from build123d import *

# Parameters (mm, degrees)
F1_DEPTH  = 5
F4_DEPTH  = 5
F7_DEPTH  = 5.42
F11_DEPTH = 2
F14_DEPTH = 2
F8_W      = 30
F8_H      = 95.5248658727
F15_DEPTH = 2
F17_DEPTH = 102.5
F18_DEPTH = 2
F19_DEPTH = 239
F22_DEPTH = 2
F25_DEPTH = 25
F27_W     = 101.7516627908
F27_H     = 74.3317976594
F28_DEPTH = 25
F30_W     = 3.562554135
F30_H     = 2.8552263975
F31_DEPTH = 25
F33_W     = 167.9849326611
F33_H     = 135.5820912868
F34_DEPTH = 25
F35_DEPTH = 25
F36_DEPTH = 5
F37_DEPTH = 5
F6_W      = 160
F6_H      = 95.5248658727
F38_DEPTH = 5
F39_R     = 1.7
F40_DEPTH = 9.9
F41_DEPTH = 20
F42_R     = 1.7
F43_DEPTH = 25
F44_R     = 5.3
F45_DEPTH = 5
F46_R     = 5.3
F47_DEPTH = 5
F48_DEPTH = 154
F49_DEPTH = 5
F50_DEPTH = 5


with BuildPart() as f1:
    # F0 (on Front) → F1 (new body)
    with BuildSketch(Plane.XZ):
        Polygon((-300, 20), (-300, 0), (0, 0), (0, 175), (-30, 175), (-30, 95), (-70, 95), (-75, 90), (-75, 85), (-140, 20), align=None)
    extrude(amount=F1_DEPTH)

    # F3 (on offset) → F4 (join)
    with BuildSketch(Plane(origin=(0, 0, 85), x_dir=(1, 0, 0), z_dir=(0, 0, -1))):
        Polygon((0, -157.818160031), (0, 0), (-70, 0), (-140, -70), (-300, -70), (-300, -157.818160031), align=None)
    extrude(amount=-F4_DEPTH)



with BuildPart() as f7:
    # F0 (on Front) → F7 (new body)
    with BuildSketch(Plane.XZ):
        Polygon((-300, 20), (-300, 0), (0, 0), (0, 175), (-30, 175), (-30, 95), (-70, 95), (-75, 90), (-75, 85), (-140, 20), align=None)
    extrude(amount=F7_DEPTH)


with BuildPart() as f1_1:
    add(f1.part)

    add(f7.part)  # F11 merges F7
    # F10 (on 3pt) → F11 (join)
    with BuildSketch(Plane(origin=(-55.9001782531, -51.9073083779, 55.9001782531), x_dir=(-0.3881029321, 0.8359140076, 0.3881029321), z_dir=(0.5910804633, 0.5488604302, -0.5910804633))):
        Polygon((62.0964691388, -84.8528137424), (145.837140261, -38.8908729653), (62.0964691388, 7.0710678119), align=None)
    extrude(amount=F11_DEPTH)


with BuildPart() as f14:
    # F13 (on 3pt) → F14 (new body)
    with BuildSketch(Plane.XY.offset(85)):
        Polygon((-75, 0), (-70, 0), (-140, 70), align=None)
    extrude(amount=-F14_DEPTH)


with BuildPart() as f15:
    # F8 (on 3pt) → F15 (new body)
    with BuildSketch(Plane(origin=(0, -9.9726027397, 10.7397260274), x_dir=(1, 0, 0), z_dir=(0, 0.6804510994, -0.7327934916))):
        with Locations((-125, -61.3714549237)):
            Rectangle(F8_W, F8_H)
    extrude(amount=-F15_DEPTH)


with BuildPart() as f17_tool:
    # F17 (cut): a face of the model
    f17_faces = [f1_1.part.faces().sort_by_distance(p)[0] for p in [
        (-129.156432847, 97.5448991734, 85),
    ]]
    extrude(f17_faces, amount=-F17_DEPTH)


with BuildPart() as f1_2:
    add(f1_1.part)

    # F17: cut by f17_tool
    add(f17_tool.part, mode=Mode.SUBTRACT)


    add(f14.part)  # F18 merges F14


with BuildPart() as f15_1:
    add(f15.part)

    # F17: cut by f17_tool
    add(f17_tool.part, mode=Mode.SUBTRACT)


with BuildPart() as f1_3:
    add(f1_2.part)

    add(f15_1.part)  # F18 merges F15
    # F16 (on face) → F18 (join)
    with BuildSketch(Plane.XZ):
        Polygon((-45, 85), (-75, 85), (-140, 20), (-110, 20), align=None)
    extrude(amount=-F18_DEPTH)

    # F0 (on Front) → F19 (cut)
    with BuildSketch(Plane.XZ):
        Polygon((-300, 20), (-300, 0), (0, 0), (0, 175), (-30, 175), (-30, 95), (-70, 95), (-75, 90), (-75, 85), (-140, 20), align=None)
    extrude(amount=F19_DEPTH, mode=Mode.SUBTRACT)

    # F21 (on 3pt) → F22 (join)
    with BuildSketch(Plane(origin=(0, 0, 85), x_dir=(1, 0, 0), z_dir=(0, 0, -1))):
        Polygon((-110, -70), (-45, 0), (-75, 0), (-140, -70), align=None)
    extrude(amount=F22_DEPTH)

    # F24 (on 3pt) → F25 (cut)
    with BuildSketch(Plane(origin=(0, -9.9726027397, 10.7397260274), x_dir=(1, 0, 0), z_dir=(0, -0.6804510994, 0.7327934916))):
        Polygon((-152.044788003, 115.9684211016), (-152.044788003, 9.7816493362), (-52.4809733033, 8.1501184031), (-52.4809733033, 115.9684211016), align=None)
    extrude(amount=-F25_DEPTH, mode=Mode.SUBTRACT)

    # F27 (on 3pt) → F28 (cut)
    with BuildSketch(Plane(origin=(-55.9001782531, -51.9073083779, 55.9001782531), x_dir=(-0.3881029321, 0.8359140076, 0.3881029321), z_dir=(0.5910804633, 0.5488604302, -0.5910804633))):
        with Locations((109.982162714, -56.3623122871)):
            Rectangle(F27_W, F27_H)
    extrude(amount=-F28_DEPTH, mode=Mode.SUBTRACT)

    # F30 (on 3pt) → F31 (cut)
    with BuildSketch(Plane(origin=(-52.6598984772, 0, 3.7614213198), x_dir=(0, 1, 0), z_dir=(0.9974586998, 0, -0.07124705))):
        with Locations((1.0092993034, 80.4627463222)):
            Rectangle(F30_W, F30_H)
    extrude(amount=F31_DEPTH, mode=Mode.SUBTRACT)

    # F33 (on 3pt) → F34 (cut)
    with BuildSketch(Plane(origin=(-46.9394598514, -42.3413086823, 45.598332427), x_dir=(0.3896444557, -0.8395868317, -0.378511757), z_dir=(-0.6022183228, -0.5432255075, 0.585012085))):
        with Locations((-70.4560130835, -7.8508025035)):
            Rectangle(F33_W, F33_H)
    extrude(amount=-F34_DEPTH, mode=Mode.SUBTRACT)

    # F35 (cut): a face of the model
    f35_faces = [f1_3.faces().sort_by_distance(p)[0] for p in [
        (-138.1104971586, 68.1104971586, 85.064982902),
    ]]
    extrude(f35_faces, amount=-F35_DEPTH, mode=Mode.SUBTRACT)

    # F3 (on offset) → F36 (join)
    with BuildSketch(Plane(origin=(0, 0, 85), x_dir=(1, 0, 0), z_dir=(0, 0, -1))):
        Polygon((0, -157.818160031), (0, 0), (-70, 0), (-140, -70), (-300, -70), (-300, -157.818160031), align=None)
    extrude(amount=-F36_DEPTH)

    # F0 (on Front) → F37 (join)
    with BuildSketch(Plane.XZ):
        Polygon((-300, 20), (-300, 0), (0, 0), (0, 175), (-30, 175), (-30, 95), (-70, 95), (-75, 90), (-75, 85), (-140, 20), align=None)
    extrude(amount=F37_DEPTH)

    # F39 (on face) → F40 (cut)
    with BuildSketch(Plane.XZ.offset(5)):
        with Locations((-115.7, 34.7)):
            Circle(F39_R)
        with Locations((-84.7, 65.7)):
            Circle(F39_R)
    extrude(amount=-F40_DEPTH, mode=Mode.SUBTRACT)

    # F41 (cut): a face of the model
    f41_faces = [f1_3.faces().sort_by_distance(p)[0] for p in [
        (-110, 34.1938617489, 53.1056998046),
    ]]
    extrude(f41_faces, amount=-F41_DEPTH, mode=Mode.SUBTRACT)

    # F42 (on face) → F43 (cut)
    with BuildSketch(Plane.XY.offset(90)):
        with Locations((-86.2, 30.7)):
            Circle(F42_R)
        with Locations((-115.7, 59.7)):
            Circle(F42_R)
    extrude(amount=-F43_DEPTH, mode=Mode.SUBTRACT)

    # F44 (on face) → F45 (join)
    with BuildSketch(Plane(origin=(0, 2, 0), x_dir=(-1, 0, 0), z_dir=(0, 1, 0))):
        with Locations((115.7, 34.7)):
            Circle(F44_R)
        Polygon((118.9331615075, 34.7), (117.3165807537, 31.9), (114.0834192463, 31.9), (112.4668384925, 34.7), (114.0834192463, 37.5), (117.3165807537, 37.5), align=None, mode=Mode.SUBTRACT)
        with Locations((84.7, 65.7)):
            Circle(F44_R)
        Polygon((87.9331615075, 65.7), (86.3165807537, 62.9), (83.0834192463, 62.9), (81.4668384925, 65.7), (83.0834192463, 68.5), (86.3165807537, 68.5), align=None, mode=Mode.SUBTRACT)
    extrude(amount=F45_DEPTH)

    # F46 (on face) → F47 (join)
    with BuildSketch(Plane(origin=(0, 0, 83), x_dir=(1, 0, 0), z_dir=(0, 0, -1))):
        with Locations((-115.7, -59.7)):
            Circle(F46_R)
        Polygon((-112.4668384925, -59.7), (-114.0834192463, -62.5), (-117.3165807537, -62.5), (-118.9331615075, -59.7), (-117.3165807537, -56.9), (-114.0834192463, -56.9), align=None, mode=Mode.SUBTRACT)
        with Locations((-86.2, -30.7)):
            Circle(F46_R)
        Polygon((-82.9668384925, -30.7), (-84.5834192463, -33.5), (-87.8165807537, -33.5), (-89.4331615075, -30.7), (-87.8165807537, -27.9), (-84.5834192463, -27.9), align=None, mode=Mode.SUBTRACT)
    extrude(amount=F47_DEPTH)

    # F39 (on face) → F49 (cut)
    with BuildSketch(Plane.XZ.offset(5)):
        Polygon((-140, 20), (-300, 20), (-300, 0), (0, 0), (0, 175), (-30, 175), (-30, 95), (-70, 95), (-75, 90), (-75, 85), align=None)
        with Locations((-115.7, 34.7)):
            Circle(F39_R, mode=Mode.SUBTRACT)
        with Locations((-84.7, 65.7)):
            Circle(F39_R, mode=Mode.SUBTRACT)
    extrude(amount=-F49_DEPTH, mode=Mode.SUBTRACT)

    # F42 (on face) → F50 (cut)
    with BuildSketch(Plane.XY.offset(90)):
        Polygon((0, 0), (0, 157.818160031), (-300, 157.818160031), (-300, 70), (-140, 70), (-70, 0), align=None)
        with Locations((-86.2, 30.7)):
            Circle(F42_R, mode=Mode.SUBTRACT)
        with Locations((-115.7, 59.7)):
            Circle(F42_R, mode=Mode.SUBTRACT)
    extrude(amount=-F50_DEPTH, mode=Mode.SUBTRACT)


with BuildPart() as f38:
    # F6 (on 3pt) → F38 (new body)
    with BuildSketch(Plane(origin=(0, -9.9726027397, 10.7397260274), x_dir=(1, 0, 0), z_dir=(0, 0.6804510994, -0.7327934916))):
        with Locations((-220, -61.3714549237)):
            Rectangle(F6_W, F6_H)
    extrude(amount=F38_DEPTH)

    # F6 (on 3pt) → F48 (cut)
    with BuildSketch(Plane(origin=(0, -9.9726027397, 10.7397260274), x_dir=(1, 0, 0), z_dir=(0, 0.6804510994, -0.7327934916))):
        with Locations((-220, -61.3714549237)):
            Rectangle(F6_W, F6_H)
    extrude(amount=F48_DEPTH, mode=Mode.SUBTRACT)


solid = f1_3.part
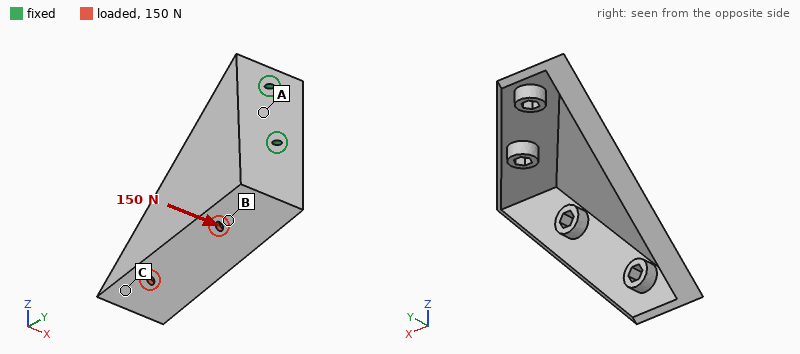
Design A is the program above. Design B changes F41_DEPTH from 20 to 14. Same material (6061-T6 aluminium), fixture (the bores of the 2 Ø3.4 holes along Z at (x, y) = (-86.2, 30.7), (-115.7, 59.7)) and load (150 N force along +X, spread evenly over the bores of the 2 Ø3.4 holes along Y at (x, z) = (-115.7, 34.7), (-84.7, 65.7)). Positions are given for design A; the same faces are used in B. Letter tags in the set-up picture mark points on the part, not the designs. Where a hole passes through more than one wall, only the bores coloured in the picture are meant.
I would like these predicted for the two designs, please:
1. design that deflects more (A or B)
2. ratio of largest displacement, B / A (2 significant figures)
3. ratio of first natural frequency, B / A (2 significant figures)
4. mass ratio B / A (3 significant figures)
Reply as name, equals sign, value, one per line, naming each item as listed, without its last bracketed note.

design that deflects more = A
ratio of largest displacement, B / A = 0.72
ratio of first natural frequency, B / A = 1.1
mass ratio B / A = 1.06
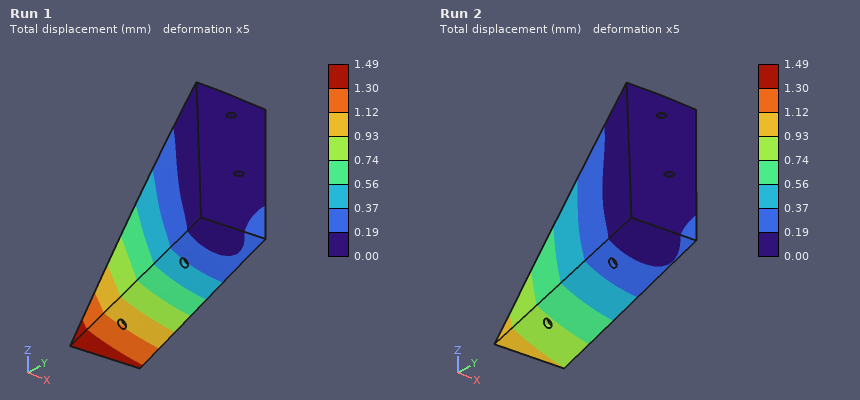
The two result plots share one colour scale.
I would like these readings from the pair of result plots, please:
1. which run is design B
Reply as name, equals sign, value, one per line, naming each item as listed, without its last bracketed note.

which run is design B = Run 2
